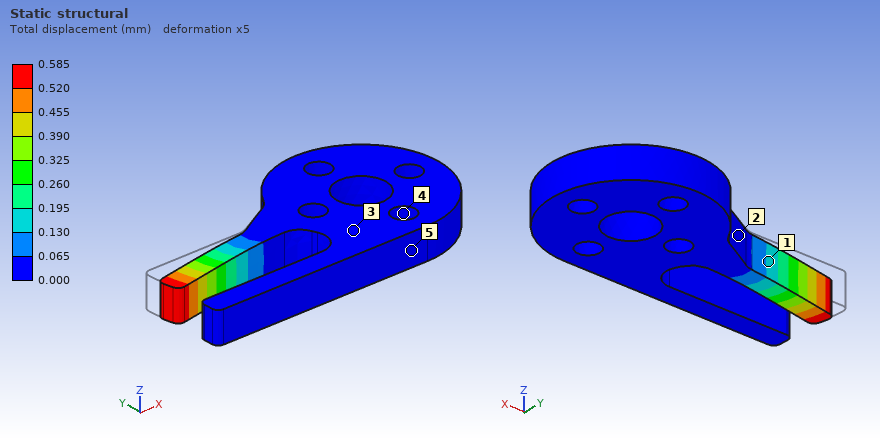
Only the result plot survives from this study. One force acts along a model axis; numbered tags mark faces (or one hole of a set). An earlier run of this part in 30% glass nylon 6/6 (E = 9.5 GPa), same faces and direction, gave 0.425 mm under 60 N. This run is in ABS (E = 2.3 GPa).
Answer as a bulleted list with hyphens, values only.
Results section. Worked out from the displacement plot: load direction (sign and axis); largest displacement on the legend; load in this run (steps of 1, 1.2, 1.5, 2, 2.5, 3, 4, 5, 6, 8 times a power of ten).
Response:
- -Y
- 0.585 mm
- 20 N
